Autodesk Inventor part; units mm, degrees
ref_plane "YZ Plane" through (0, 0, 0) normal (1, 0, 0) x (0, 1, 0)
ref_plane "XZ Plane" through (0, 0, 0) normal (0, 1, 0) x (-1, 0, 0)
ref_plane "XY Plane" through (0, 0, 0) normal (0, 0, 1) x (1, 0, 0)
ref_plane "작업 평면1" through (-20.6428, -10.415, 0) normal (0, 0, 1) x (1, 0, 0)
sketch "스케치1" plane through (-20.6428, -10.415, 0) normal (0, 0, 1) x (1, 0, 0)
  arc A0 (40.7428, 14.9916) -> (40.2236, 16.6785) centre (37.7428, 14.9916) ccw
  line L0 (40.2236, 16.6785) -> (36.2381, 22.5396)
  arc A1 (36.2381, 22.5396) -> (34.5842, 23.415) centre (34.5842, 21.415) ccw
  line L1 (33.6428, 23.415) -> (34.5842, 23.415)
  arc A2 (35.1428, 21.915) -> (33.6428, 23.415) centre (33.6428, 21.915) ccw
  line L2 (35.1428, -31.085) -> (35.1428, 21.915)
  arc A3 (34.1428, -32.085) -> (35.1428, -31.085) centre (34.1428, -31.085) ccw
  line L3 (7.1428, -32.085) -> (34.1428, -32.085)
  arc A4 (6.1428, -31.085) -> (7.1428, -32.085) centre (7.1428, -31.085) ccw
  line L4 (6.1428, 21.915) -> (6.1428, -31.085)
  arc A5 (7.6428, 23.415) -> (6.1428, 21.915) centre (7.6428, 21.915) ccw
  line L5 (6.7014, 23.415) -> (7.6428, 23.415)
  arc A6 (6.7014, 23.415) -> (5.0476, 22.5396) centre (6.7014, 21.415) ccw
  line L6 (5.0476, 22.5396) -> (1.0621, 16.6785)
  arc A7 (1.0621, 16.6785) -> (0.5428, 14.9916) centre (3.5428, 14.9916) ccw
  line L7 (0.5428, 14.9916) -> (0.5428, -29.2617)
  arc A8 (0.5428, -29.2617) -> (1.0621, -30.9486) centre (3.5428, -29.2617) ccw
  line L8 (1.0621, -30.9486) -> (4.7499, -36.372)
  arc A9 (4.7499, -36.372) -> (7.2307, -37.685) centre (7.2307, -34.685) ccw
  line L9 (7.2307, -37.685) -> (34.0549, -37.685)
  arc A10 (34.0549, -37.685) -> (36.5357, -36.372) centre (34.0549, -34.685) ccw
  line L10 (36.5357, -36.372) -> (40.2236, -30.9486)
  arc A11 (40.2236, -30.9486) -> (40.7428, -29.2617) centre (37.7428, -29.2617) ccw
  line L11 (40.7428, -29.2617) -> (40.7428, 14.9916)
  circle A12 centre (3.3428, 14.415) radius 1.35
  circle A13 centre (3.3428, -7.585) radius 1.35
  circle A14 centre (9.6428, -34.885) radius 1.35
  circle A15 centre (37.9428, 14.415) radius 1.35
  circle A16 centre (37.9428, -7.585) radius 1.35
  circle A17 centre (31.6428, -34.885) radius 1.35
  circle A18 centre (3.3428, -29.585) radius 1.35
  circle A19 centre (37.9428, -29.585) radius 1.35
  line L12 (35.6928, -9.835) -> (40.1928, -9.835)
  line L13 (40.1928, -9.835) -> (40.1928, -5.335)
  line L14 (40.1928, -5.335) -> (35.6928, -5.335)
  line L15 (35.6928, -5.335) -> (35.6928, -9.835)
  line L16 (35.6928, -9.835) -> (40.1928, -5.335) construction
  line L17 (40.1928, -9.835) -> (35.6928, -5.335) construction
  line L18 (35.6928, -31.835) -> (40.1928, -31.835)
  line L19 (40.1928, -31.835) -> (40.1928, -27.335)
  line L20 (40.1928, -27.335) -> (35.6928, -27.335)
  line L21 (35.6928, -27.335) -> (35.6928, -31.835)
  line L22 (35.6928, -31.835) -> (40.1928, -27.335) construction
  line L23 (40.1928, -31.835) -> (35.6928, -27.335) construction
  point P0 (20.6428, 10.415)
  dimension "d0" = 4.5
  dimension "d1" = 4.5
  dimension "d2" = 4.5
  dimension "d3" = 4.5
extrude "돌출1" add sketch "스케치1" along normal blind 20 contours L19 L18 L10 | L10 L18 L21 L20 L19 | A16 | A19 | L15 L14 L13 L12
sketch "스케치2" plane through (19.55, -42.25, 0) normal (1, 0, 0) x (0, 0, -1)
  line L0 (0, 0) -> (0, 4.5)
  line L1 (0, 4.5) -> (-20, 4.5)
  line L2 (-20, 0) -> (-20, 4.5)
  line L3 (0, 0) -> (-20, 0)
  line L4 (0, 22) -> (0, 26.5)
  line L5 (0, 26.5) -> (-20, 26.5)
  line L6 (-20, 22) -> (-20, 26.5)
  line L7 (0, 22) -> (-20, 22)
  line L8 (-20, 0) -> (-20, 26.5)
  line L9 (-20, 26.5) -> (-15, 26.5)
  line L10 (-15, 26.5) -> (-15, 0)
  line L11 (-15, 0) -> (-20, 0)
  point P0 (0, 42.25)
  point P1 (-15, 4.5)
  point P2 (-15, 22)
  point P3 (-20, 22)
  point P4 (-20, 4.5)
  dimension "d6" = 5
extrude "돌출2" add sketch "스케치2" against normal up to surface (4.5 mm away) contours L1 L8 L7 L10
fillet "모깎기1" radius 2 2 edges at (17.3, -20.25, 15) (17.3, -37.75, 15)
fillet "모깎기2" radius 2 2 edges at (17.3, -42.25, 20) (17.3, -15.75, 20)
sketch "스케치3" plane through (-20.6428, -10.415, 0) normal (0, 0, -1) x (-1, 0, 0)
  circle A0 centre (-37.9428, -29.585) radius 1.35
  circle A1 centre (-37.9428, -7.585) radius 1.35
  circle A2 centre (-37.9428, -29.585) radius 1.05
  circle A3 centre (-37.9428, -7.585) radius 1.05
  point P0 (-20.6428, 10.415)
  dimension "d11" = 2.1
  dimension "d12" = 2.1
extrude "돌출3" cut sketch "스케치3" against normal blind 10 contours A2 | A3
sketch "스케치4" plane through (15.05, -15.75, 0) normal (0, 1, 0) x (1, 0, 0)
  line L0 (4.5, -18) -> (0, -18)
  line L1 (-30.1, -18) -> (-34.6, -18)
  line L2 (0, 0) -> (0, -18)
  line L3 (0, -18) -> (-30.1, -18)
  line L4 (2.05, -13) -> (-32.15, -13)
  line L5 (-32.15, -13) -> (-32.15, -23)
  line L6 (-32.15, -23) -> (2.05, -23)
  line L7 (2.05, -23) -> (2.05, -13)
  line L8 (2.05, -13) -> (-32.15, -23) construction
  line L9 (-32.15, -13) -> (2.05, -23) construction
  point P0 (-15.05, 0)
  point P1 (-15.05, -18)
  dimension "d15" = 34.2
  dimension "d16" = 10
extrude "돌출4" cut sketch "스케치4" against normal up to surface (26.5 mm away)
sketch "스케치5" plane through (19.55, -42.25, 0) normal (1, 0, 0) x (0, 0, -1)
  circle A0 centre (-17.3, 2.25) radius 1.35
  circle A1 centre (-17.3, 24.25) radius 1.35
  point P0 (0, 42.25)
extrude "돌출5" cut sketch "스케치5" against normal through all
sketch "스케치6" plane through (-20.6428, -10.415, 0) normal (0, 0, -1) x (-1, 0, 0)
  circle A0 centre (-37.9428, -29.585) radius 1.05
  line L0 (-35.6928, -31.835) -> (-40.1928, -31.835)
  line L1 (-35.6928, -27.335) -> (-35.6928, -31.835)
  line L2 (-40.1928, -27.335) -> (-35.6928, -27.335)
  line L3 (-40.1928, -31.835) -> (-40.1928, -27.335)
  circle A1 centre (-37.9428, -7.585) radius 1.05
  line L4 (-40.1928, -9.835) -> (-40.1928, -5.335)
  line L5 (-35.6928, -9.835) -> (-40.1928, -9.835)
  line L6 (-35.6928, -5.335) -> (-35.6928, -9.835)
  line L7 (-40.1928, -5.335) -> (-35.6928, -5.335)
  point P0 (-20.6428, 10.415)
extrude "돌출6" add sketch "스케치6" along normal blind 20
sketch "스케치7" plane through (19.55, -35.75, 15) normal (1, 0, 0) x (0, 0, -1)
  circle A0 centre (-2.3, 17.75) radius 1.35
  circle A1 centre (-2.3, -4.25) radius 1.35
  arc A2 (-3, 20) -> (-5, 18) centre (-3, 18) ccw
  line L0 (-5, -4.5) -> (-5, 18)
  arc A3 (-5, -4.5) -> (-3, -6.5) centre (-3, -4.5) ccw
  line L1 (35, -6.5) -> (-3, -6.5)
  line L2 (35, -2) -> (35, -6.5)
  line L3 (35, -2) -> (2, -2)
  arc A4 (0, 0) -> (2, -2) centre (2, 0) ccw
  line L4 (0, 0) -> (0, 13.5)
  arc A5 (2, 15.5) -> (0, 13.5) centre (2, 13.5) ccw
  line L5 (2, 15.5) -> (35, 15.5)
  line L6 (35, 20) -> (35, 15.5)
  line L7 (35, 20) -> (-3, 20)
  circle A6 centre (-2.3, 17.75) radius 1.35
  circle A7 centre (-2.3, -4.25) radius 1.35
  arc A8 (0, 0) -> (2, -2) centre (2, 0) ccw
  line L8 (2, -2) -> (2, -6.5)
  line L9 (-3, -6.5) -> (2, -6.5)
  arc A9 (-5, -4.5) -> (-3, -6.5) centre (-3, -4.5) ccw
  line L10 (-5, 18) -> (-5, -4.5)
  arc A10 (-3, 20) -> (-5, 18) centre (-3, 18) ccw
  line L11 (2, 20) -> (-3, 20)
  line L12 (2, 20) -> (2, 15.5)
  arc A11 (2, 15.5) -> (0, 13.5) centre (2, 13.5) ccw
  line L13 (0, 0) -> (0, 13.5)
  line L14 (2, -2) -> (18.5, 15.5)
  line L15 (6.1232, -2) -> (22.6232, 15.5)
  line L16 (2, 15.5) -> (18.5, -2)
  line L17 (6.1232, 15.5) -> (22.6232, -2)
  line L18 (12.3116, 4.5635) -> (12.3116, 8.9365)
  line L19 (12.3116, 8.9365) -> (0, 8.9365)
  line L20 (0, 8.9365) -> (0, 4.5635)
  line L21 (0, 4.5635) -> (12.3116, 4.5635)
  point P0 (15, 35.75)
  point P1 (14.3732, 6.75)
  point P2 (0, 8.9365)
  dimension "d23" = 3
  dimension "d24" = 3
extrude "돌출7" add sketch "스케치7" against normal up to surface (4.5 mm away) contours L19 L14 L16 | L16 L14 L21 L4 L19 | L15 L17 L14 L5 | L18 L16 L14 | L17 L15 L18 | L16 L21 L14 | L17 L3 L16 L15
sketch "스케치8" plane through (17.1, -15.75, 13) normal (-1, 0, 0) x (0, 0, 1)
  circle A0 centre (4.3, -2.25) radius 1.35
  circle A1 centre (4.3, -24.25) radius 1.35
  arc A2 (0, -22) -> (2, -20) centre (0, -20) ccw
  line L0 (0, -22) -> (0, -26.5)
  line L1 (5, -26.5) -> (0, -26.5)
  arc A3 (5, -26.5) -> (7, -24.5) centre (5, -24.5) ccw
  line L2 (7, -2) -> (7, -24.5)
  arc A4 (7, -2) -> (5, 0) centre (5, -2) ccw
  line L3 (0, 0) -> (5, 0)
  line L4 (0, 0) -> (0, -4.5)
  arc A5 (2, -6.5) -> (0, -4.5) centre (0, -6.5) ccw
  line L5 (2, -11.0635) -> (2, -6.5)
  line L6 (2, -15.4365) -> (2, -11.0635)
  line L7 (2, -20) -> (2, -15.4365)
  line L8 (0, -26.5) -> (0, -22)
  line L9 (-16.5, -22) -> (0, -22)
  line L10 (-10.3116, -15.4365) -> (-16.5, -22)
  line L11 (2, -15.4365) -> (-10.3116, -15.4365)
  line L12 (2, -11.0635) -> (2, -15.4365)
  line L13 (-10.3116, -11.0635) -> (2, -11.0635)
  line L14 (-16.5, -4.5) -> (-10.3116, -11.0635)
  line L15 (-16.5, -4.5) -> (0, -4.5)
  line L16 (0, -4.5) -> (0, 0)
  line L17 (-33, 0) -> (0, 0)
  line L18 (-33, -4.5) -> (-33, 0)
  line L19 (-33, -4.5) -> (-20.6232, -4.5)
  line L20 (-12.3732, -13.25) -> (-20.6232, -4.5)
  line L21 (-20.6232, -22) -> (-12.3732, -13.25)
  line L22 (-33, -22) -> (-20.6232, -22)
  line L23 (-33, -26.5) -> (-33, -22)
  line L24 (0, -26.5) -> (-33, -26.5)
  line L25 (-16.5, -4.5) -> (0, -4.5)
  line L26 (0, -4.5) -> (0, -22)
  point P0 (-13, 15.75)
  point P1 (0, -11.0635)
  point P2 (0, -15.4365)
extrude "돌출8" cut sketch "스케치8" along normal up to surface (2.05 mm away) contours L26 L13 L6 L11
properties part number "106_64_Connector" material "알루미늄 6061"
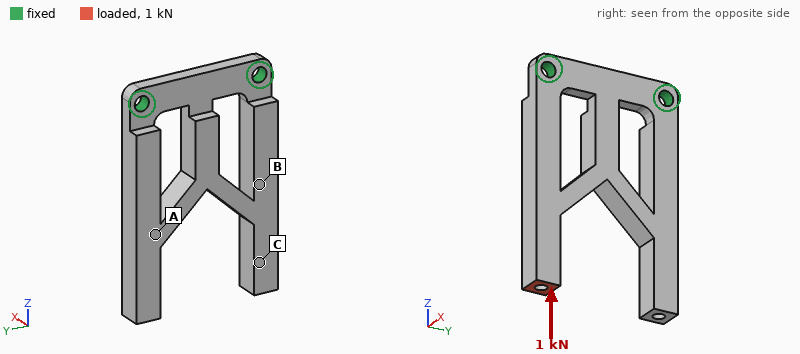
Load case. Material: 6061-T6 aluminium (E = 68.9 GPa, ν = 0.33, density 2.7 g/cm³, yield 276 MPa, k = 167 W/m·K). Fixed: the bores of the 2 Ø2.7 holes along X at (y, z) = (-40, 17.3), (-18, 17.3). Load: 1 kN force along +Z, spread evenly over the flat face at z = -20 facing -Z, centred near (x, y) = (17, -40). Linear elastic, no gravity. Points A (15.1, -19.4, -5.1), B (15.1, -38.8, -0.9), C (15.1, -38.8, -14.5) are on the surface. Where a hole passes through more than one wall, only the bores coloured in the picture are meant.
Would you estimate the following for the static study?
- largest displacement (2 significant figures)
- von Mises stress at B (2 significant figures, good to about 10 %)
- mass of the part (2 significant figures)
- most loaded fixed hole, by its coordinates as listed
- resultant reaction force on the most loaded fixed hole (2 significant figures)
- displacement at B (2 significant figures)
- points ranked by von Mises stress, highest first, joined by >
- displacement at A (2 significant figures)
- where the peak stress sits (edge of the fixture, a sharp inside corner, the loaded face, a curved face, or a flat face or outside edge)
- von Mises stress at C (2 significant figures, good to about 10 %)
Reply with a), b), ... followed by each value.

a) 0.20 mm
b) 45 MPa
c) 5.4 g
d) (-40, 17.3)
e) 990 N
f) 0.093 mm
g) C > B > A
h) 0.061 mm
i) a flat face or outside edge
j) 60 MPa
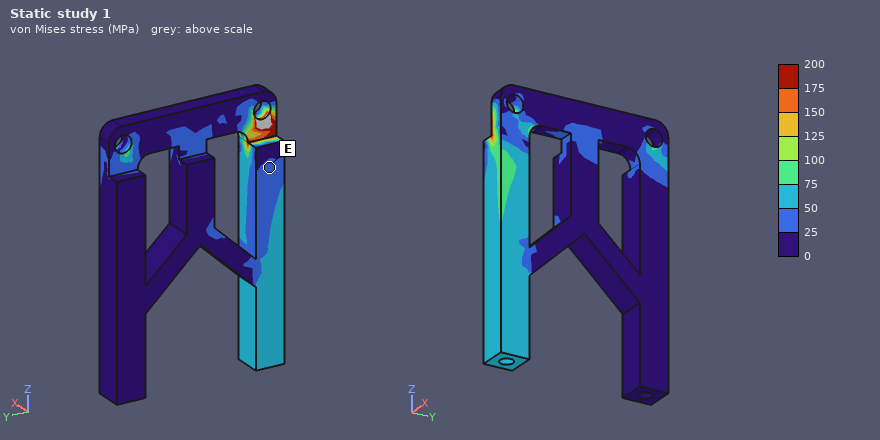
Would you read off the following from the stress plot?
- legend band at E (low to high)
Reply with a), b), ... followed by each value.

a) 25 to 50 MPa
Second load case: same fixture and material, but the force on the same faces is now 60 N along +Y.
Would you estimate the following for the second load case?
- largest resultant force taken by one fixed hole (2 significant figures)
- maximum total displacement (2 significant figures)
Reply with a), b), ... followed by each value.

a) 110 N
b) 72 µm
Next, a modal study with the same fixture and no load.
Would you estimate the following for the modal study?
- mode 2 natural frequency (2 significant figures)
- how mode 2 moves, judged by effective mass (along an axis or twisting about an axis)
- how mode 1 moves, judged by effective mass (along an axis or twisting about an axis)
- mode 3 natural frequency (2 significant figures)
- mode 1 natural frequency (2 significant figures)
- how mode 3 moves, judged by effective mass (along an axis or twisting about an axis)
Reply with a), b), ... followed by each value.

a) 3500 Hz
b) twisting about Z
c) along X
d) 6400 Hz
e) 1800 Hz
f) along Y
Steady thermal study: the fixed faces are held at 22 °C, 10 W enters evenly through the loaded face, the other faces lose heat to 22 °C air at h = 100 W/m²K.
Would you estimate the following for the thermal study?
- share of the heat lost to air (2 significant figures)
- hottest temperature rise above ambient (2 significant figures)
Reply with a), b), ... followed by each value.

a) 40 %
b) 78 K
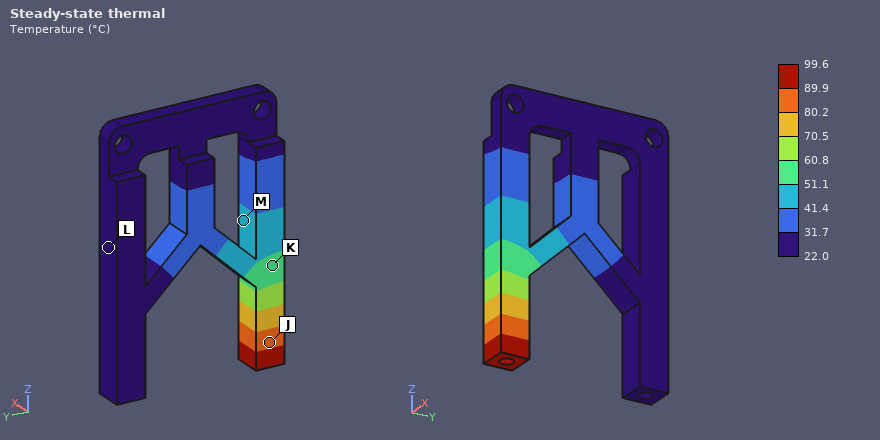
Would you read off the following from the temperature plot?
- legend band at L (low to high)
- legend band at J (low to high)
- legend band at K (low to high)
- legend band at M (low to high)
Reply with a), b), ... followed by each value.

a) 22.0 to 31.7 °C
b) 80.2 to 89.9 °C
c) 51.1 to 60.8 °C
d) 41.4 to 51.1 °C
